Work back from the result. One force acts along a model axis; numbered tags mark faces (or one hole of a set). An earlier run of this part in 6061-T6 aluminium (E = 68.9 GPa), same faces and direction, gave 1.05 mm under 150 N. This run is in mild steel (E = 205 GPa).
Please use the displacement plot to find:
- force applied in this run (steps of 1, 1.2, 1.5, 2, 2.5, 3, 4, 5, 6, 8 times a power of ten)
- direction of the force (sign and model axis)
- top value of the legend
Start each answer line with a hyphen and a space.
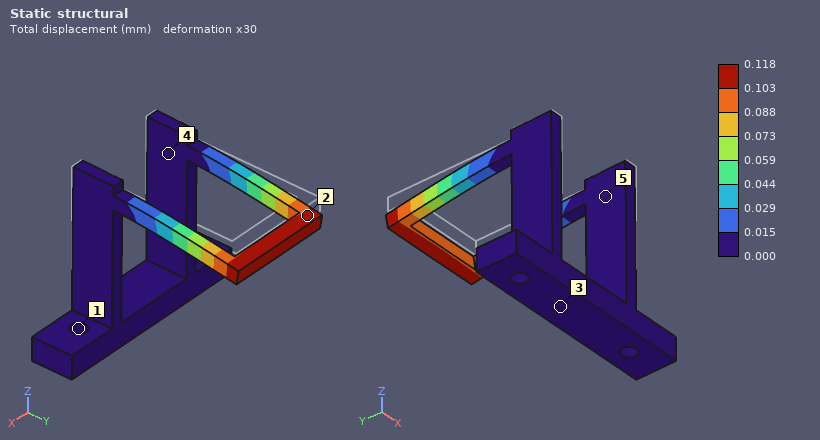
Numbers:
- 50 N
- -Z
- 0.118 mm
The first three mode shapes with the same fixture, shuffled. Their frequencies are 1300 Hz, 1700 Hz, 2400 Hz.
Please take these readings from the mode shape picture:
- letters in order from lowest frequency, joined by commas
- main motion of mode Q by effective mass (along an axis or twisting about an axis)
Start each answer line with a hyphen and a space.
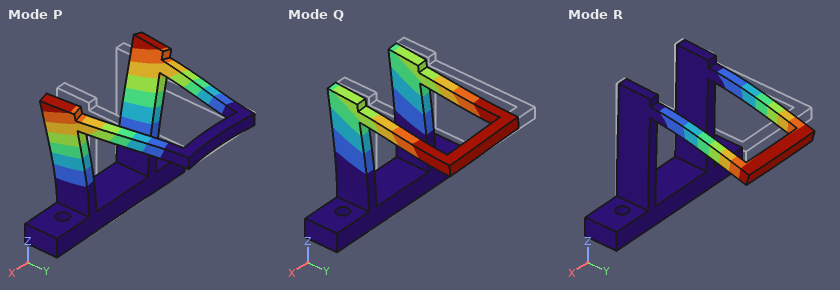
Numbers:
- Q, R, P
- along X
